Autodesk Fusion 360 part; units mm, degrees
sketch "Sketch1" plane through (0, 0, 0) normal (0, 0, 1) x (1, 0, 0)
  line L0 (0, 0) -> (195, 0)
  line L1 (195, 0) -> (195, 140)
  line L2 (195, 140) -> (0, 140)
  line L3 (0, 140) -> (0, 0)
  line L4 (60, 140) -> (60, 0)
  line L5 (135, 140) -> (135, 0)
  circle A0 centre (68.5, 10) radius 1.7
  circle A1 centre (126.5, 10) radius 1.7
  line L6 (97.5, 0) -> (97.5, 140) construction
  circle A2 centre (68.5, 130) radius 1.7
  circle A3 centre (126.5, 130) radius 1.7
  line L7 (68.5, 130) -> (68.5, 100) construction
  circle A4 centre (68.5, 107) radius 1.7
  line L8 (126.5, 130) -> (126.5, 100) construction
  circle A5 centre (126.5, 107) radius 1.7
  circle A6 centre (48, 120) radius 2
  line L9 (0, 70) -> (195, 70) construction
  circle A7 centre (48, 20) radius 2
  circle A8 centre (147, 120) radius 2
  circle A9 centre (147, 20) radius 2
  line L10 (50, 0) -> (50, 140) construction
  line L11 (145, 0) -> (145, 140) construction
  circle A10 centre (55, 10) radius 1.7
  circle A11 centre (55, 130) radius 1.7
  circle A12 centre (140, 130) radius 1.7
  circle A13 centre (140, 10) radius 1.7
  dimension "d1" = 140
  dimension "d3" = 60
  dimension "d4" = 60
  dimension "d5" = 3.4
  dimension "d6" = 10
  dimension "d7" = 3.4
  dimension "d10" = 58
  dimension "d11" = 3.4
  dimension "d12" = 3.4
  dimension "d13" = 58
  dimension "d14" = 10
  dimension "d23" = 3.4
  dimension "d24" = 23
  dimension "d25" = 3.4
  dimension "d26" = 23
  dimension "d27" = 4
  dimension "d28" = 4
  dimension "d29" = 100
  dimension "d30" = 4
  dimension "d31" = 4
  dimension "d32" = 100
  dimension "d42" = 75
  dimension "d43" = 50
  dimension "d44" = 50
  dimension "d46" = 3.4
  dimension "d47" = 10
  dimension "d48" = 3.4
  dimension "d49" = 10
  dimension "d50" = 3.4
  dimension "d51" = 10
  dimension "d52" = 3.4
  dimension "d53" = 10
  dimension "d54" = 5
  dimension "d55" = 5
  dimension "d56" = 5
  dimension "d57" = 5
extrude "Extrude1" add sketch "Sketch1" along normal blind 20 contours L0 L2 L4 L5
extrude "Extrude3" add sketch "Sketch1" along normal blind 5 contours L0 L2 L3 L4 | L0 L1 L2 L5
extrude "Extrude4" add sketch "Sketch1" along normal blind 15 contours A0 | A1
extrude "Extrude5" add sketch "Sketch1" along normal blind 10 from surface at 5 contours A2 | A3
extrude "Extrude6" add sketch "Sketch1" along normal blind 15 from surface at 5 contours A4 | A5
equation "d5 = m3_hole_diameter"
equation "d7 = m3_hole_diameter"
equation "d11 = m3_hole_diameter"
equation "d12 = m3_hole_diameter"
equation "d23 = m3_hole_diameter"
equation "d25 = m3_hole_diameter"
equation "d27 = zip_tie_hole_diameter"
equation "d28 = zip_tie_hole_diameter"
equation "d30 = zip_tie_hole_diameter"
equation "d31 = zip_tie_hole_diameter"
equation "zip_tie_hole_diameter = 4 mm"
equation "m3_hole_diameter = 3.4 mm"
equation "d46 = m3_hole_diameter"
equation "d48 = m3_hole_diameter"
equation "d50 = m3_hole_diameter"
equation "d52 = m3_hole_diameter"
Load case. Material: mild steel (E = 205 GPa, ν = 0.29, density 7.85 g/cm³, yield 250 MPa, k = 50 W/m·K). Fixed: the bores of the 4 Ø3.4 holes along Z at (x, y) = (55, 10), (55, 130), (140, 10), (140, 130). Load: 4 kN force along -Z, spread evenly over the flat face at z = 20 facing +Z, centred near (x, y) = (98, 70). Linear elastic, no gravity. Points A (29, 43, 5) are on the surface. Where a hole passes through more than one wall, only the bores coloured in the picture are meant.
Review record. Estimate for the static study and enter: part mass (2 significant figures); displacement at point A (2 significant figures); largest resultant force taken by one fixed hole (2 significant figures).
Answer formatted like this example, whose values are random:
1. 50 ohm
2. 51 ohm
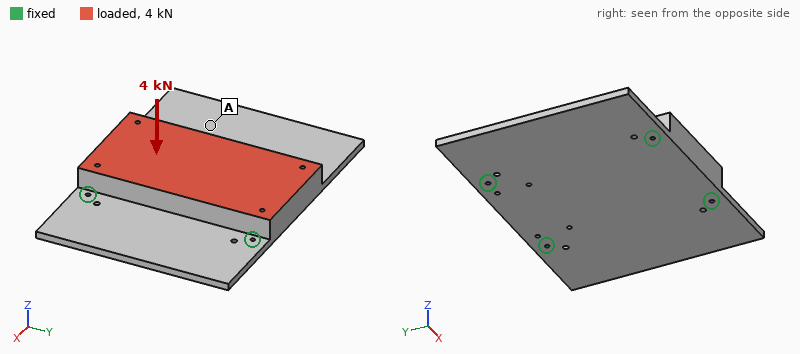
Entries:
1. 2.3 kg
2. 4.6 µm
3. 1.4 kN
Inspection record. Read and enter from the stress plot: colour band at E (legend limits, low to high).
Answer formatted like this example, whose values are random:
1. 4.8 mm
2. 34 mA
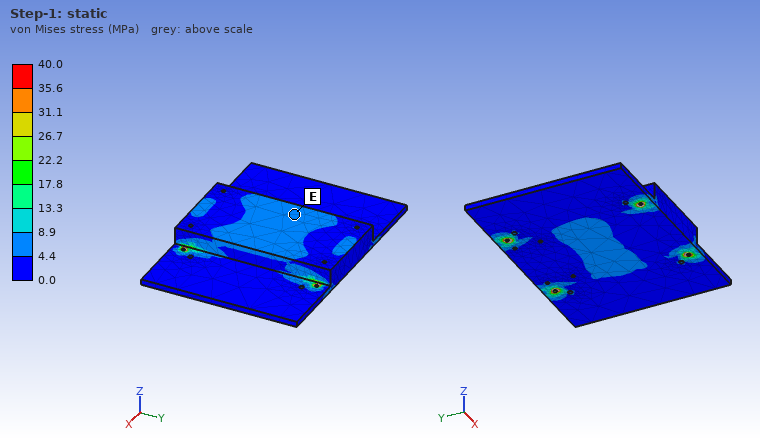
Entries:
1. 4.4 to 8.9 MPa
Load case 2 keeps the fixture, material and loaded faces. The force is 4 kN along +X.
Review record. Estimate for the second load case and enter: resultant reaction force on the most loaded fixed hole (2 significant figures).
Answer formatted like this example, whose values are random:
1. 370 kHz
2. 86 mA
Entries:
1. 1.1 kN
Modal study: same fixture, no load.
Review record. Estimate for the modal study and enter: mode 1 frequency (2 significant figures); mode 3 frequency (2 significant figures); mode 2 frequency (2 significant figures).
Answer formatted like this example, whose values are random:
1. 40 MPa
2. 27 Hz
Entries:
1. 1100 Hz
2. 1700 Hz
3. 1100 Hz
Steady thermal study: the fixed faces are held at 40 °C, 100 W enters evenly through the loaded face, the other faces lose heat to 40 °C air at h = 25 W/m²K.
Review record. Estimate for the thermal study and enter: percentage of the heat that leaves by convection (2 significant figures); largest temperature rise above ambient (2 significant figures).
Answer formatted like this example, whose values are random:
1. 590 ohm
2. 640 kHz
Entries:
1. 34 %
2. 43 K
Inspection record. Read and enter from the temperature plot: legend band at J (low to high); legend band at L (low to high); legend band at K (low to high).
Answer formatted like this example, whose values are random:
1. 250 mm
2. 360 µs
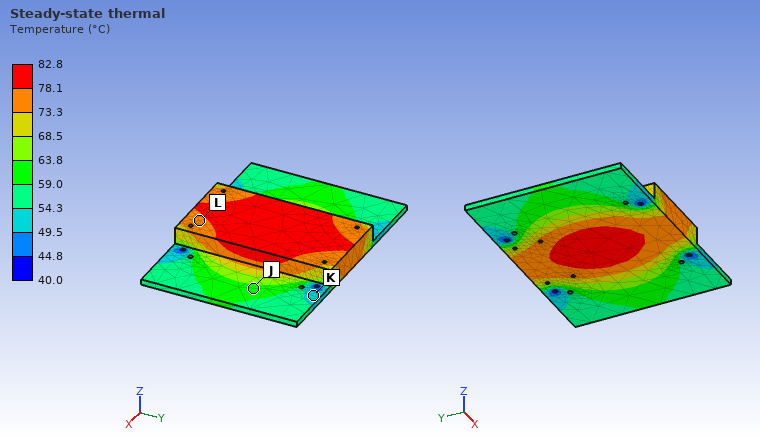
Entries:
1. 59.0 to 63.8 °C
2. 73.3 to 78.1 °C
3. 49.5 to 54.3 °C
